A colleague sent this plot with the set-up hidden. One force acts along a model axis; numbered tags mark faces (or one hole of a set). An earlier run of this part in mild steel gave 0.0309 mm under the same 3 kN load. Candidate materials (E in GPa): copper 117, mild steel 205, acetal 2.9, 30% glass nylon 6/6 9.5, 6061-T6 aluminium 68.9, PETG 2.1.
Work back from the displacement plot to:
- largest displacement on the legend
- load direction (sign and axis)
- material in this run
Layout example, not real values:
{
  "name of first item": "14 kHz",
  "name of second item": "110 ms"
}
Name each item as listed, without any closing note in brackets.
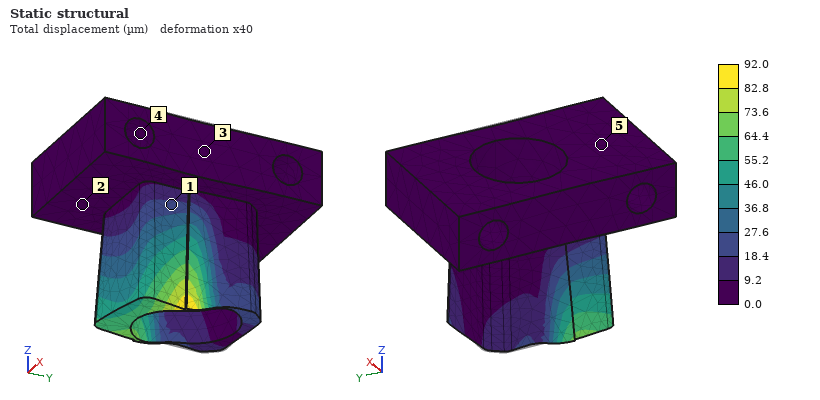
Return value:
{
  "largest displacement on the legend": "92.0 µm",
  "load direction": "-X",
  "material in this run": "6061-T6 aluminium"
}
